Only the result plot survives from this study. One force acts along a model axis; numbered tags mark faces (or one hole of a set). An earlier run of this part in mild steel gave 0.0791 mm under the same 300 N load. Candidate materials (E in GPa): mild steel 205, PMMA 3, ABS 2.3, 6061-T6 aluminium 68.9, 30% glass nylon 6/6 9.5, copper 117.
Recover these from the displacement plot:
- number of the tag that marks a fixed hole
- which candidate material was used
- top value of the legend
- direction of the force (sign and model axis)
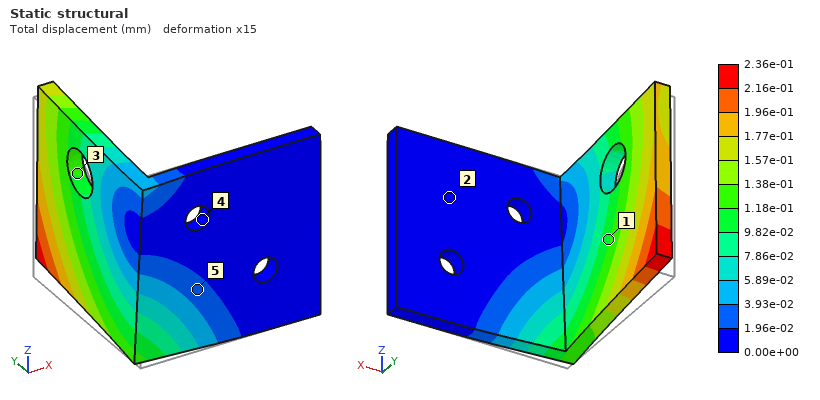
4
6061-T6 aluminium
2.36e-01 mm
+Z
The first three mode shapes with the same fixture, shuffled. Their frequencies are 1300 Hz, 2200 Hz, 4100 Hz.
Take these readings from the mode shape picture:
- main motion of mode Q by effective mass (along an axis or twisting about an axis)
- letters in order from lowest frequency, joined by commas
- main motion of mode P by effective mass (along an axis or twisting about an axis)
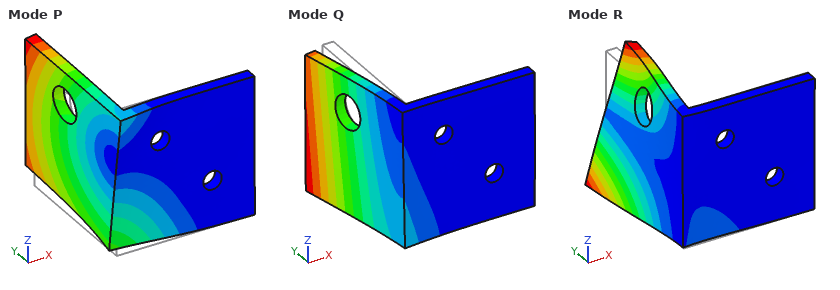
along X
Q, P, R
along Z
